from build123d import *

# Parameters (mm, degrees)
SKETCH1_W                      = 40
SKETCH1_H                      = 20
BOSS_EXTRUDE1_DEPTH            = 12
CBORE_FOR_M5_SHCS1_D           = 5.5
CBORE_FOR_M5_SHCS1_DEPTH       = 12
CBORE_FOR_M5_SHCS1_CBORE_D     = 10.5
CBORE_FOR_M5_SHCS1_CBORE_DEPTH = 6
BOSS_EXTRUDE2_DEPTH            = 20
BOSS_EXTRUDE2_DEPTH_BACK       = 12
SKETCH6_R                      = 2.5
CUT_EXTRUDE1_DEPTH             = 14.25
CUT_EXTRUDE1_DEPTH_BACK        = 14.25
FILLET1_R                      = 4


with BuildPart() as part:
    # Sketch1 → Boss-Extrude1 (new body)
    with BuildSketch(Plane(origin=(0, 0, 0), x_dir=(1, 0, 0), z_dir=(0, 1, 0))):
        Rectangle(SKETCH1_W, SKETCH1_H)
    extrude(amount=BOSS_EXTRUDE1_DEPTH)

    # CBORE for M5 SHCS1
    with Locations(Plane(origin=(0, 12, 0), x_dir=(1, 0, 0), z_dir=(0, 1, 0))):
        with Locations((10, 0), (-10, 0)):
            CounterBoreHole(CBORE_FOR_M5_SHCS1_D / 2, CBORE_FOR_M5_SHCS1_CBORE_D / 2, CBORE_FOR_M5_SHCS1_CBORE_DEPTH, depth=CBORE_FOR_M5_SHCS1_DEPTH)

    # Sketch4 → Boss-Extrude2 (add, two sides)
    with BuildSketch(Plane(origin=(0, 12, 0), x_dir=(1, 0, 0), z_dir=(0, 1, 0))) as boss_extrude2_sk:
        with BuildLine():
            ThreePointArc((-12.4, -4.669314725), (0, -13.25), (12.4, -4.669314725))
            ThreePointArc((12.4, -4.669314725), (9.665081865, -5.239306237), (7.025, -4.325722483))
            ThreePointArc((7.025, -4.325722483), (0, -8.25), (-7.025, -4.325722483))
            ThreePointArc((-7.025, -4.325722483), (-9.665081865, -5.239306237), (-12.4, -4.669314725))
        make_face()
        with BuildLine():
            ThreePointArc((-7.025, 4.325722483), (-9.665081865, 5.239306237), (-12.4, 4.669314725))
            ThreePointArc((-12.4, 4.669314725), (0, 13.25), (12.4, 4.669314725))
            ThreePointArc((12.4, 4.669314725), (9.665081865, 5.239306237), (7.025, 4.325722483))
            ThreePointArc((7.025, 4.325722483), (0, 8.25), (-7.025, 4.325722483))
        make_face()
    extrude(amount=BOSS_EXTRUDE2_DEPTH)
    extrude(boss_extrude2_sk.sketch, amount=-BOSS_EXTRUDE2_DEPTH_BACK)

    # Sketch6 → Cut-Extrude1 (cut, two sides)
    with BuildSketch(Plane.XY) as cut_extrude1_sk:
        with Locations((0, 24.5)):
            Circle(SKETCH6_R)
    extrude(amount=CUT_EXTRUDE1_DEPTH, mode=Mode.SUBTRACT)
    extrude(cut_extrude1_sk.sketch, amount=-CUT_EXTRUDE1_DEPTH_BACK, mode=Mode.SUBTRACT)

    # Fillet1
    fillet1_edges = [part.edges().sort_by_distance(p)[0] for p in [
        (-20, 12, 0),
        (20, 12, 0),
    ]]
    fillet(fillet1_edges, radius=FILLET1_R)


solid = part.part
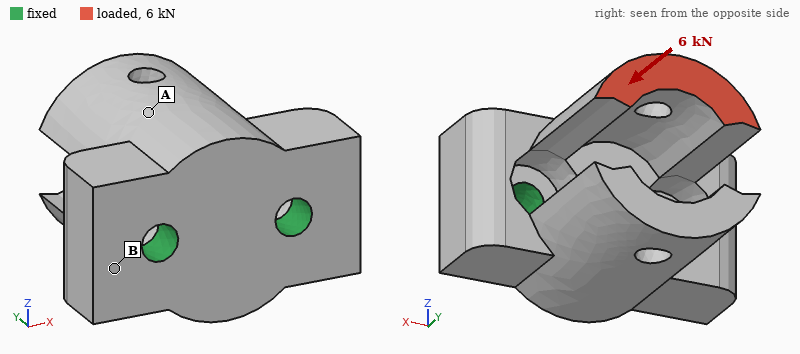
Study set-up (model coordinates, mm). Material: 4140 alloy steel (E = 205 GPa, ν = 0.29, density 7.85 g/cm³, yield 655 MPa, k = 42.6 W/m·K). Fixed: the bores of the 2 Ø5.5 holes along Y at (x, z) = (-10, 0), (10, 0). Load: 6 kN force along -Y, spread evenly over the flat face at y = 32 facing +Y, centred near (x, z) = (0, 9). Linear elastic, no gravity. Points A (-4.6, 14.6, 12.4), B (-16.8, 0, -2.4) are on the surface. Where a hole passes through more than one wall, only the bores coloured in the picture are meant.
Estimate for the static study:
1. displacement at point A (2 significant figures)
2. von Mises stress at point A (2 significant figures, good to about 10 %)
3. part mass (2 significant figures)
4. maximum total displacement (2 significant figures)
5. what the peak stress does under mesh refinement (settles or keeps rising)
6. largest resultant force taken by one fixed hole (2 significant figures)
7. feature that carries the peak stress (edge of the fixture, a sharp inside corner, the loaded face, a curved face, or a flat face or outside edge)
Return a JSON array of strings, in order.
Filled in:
["19 µm", "58 MPa", "110 g", "43 µm", "keeps rising", "3.1 kN", "edge of the fixture"]
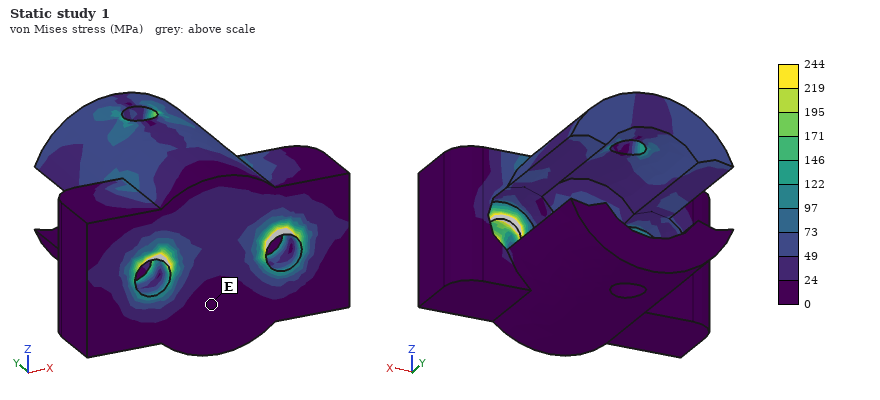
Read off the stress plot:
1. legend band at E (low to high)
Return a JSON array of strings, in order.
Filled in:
["0 to 24 MPa"]
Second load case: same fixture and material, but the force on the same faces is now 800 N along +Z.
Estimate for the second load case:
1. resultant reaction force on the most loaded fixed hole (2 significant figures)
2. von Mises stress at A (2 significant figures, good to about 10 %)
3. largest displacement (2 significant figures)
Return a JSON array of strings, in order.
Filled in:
["470 N", "97 MPa", "61 µm"]
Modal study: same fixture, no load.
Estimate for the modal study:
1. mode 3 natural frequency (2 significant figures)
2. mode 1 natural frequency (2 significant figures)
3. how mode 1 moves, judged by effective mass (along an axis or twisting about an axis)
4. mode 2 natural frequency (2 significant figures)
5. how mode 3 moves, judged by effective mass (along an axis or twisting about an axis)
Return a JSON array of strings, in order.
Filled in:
["14 kHz", "6600 Hz", "along Z", "8700 Hz", "along X"]
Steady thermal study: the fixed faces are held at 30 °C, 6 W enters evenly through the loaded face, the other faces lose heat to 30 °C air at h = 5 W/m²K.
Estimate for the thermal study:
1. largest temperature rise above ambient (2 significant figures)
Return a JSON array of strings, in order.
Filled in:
["35 K"]
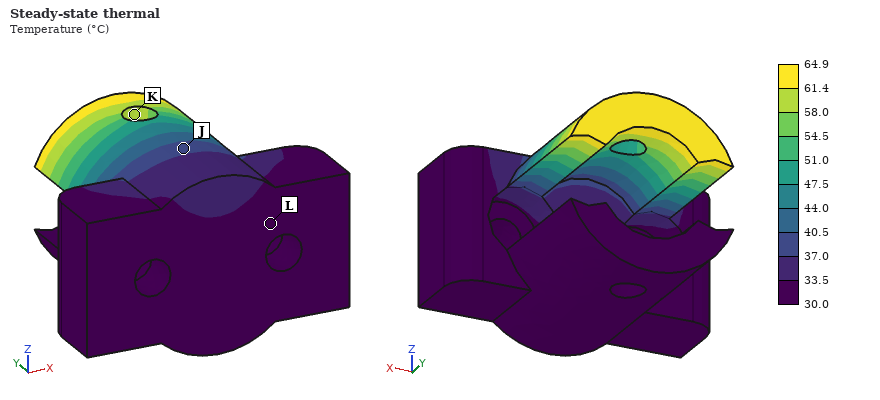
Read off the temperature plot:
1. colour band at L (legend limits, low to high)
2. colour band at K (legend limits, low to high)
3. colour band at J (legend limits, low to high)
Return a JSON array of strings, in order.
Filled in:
["30.0 to 33.5 °C", "58.0 to 61.4 °C", "37.0 to 40.5 °C"]
